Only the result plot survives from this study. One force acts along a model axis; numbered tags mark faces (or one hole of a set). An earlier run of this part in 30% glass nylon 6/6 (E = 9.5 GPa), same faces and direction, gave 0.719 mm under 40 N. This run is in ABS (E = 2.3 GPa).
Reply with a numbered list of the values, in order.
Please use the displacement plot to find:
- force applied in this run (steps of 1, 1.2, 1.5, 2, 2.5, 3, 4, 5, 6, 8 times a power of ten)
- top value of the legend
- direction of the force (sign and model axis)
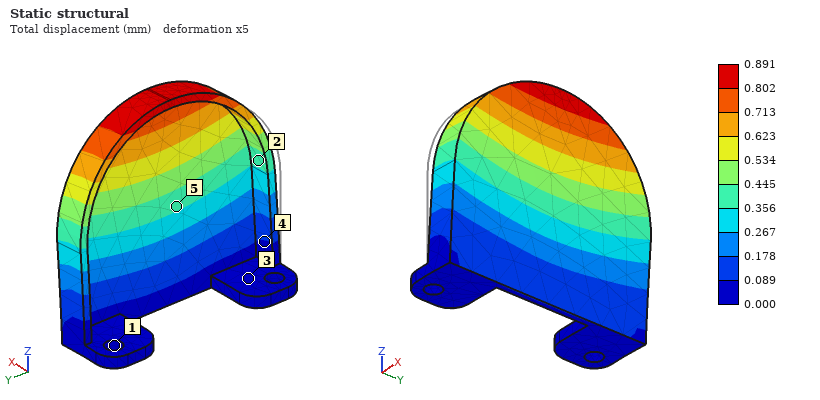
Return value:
1. 12 N
2. 0.891 mm
3. +X
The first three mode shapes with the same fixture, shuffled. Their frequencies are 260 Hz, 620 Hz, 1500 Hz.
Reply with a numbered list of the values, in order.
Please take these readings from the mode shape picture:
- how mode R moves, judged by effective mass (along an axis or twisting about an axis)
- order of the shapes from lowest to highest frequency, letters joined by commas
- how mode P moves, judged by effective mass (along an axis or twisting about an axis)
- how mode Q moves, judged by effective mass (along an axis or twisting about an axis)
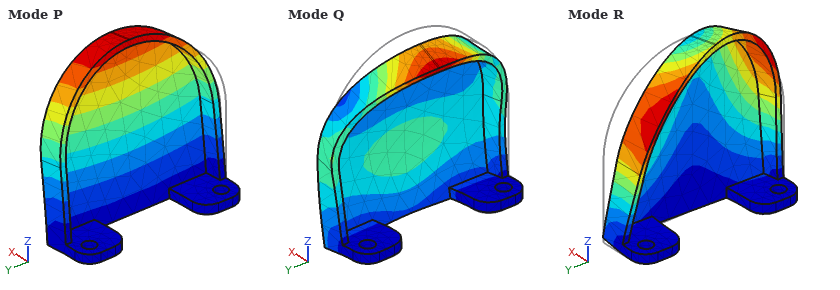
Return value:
1. along Y
2. P, R, Q
3. along X
4. along Z
